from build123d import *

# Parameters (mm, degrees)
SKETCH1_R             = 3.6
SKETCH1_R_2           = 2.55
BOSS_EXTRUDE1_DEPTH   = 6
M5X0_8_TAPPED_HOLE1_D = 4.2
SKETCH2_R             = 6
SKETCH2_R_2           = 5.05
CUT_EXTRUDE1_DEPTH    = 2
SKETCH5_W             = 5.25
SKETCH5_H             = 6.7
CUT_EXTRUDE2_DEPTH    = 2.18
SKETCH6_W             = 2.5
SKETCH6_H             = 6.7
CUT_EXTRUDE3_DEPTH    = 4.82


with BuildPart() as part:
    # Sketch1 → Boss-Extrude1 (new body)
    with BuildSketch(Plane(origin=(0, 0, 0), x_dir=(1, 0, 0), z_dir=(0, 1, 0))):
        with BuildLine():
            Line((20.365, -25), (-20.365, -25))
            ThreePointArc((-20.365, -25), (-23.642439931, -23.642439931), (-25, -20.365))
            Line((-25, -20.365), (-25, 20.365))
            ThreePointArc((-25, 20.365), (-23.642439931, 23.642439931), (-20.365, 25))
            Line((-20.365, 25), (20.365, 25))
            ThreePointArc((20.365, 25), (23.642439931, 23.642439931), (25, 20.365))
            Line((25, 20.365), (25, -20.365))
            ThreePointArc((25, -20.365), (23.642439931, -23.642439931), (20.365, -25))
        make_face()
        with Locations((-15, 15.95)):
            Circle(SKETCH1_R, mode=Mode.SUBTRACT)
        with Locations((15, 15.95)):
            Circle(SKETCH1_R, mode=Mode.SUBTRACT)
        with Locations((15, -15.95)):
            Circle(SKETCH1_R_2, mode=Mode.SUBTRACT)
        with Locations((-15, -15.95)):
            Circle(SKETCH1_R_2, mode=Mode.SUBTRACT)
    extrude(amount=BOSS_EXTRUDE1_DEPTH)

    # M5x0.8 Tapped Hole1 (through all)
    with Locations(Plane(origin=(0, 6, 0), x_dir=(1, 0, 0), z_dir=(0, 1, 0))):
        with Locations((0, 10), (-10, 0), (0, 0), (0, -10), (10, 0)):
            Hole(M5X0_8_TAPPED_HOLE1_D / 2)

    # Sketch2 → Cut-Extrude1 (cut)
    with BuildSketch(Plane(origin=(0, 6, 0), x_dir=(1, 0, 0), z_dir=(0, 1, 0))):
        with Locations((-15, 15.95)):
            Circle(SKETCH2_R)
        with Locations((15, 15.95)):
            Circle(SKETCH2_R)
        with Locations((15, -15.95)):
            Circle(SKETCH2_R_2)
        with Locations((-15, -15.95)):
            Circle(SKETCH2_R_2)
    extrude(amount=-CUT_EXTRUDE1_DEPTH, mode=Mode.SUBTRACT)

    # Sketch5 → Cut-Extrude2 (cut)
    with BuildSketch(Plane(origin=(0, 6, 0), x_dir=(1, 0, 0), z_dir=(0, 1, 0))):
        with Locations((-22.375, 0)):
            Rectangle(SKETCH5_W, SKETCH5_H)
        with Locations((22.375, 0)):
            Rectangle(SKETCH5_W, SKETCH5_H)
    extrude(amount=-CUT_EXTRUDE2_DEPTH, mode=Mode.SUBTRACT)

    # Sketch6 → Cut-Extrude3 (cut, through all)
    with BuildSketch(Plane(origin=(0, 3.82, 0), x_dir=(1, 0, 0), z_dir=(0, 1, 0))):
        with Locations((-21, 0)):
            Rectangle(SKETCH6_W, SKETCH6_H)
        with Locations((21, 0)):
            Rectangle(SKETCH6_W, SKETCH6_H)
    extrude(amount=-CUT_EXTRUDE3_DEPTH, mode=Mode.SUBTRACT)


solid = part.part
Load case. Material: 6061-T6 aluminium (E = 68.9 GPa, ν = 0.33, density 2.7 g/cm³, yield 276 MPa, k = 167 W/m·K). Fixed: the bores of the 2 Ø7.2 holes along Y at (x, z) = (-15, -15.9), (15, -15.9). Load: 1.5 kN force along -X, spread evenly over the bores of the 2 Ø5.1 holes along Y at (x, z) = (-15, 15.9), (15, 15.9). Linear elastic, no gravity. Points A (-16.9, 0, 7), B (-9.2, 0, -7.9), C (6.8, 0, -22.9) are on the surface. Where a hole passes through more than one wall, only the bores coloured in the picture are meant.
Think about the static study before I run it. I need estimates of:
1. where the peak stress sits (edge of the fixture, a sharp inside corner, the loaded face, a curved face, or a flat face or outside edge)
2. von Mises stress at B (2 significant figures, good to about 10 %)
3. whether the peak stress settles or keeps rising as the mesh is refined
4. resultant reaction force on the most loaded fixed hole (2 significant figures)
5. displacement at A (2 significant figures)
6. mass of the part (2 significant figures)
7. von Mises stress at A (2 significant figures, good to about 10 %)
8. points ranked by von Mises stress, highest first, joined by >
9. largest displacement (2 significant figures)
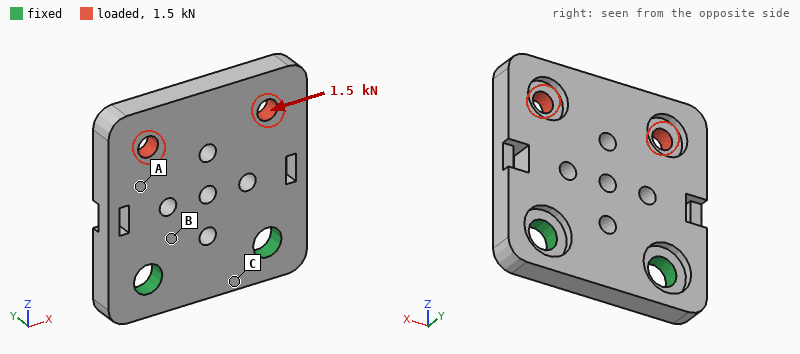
edge of the fixture
23 MPa
keeps rising
1.5 kN
14 µm
35 g
12 MPa
B > A > C
27 µm
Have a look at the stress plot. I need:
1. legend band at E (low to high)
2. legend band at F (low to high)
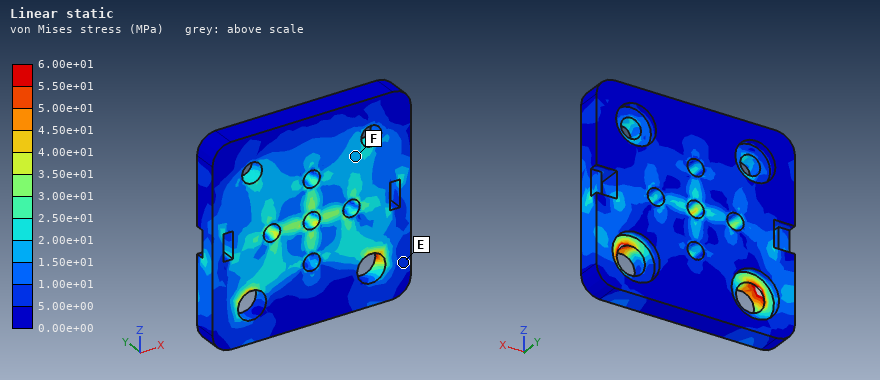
5.00e+00 to 1.00e+01 MPa
1.50e+01 to 2.00e+01 MPa
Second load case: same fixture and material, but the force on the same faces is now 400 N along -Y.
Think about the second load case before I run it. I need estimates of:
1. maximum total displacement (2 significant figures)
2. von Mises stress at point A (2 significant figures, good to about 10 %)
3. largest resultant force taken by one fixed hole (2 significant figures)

0.14 mm
14 MPa
200 N
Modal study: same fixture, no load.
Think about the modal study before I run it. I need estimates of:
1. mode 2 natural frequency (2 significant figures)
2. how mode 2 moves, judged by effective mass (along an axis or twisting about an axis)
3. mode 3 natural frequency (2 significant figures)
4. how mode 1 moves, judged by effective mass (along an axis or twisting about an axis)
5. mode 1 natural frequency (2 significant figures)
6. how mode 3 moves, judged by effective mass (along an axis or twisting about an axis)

5400 Hz
twisting about Z
12 kHz
along Y
2600 Hz
along X
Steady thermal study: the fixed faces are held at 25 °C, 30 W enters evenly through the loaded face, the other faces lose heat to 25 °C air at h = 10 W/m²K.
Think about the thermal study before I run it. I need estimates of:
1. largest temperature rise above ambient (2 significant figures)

27 K
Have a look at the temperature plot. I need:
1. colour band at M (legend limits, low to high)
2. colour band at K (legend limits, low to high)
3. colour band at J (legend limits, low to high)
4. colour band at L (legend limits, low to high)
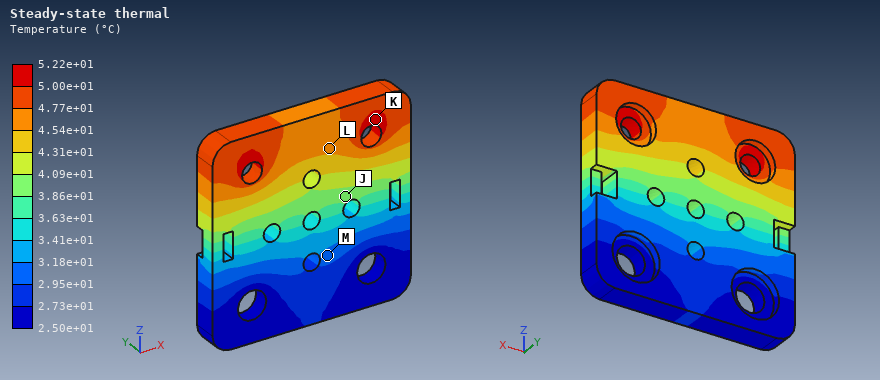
2.95e+01 to 3.18e+01 °C
5.00e+01 to 5.22e+01 °C
3.86e+01 to 4.09e+01 °C
4.54e+01 to 4.77e+01 °C
